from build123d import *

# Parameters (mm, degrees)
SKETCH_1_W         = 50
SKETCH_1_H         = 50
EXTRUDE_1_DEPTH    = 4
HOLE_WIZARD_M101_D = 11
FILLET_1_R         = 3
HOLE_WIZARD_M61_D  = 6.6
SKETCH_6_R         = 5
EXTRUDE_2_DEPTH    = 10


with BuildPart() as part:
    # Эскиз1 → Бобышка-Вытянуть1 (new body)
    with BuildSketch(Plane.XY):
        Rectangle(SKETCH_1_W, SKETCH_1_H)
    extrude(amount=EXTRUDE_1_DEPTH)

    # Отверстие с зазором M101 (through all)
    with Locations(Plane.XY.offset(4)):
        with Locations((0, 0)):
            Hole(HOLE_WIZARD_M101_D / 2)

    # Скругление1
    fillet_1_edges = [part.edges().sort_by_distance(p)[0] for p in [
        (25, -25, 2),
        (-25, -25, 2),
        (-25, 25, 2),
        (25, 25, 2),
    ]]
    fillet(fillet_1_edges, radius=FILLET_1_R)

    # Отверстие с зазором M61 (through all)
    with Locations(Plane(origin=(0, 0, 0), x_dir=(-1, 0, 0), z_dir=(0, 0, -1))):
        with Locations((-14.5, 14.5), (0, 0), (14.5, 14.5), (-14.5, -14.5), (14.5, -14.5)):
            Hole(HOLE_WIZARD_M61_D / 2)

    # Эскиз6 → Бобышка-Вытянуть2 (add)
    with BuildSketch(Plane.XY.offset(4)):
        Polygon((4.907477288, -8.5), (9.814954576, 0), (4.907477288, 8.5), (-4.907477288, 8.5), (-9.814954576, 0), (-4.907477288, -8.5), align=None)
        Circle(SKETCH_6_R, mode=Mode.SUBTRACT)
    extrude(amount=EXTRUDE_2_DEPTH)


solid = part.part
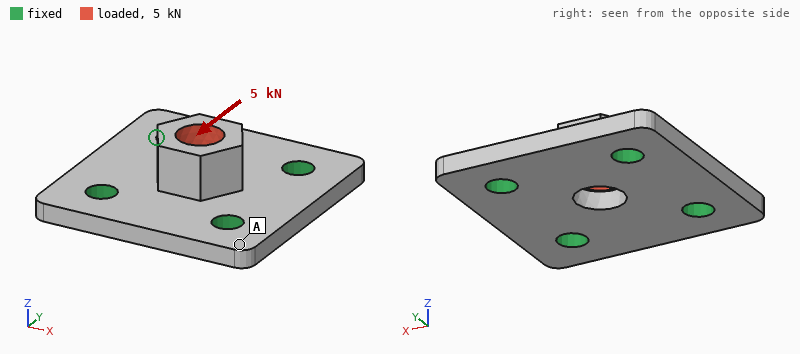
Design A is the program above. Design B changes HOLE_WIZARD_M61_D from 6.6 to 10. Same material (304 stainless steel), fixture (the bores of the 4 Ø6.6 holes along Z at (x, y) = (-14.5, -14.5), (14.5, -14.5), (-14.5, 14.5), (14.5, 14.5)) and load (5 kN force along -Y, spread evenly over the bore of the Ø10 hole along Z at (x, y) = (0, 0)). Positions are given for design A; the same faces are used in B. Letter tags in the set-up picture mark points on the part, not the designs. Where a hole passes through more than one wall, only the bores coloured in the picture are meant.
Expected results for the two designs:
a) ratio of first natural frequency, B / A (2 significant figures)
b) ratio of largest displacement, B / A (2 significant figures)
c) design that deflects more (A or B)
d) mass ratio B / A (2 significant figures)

1.3
0.82
A
0.93
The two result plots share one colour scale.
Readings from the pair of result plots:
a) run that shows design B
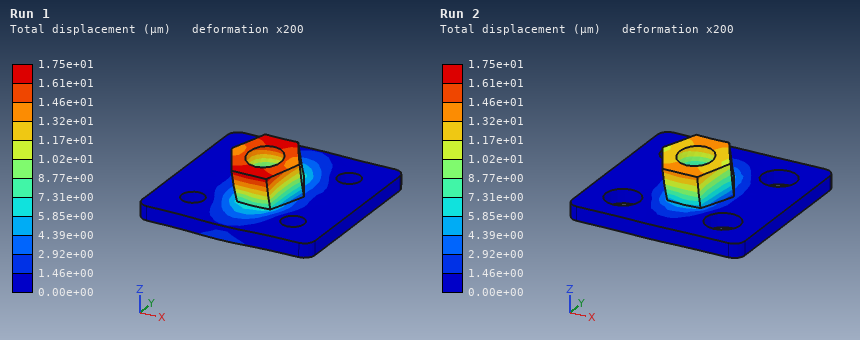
Run 2
